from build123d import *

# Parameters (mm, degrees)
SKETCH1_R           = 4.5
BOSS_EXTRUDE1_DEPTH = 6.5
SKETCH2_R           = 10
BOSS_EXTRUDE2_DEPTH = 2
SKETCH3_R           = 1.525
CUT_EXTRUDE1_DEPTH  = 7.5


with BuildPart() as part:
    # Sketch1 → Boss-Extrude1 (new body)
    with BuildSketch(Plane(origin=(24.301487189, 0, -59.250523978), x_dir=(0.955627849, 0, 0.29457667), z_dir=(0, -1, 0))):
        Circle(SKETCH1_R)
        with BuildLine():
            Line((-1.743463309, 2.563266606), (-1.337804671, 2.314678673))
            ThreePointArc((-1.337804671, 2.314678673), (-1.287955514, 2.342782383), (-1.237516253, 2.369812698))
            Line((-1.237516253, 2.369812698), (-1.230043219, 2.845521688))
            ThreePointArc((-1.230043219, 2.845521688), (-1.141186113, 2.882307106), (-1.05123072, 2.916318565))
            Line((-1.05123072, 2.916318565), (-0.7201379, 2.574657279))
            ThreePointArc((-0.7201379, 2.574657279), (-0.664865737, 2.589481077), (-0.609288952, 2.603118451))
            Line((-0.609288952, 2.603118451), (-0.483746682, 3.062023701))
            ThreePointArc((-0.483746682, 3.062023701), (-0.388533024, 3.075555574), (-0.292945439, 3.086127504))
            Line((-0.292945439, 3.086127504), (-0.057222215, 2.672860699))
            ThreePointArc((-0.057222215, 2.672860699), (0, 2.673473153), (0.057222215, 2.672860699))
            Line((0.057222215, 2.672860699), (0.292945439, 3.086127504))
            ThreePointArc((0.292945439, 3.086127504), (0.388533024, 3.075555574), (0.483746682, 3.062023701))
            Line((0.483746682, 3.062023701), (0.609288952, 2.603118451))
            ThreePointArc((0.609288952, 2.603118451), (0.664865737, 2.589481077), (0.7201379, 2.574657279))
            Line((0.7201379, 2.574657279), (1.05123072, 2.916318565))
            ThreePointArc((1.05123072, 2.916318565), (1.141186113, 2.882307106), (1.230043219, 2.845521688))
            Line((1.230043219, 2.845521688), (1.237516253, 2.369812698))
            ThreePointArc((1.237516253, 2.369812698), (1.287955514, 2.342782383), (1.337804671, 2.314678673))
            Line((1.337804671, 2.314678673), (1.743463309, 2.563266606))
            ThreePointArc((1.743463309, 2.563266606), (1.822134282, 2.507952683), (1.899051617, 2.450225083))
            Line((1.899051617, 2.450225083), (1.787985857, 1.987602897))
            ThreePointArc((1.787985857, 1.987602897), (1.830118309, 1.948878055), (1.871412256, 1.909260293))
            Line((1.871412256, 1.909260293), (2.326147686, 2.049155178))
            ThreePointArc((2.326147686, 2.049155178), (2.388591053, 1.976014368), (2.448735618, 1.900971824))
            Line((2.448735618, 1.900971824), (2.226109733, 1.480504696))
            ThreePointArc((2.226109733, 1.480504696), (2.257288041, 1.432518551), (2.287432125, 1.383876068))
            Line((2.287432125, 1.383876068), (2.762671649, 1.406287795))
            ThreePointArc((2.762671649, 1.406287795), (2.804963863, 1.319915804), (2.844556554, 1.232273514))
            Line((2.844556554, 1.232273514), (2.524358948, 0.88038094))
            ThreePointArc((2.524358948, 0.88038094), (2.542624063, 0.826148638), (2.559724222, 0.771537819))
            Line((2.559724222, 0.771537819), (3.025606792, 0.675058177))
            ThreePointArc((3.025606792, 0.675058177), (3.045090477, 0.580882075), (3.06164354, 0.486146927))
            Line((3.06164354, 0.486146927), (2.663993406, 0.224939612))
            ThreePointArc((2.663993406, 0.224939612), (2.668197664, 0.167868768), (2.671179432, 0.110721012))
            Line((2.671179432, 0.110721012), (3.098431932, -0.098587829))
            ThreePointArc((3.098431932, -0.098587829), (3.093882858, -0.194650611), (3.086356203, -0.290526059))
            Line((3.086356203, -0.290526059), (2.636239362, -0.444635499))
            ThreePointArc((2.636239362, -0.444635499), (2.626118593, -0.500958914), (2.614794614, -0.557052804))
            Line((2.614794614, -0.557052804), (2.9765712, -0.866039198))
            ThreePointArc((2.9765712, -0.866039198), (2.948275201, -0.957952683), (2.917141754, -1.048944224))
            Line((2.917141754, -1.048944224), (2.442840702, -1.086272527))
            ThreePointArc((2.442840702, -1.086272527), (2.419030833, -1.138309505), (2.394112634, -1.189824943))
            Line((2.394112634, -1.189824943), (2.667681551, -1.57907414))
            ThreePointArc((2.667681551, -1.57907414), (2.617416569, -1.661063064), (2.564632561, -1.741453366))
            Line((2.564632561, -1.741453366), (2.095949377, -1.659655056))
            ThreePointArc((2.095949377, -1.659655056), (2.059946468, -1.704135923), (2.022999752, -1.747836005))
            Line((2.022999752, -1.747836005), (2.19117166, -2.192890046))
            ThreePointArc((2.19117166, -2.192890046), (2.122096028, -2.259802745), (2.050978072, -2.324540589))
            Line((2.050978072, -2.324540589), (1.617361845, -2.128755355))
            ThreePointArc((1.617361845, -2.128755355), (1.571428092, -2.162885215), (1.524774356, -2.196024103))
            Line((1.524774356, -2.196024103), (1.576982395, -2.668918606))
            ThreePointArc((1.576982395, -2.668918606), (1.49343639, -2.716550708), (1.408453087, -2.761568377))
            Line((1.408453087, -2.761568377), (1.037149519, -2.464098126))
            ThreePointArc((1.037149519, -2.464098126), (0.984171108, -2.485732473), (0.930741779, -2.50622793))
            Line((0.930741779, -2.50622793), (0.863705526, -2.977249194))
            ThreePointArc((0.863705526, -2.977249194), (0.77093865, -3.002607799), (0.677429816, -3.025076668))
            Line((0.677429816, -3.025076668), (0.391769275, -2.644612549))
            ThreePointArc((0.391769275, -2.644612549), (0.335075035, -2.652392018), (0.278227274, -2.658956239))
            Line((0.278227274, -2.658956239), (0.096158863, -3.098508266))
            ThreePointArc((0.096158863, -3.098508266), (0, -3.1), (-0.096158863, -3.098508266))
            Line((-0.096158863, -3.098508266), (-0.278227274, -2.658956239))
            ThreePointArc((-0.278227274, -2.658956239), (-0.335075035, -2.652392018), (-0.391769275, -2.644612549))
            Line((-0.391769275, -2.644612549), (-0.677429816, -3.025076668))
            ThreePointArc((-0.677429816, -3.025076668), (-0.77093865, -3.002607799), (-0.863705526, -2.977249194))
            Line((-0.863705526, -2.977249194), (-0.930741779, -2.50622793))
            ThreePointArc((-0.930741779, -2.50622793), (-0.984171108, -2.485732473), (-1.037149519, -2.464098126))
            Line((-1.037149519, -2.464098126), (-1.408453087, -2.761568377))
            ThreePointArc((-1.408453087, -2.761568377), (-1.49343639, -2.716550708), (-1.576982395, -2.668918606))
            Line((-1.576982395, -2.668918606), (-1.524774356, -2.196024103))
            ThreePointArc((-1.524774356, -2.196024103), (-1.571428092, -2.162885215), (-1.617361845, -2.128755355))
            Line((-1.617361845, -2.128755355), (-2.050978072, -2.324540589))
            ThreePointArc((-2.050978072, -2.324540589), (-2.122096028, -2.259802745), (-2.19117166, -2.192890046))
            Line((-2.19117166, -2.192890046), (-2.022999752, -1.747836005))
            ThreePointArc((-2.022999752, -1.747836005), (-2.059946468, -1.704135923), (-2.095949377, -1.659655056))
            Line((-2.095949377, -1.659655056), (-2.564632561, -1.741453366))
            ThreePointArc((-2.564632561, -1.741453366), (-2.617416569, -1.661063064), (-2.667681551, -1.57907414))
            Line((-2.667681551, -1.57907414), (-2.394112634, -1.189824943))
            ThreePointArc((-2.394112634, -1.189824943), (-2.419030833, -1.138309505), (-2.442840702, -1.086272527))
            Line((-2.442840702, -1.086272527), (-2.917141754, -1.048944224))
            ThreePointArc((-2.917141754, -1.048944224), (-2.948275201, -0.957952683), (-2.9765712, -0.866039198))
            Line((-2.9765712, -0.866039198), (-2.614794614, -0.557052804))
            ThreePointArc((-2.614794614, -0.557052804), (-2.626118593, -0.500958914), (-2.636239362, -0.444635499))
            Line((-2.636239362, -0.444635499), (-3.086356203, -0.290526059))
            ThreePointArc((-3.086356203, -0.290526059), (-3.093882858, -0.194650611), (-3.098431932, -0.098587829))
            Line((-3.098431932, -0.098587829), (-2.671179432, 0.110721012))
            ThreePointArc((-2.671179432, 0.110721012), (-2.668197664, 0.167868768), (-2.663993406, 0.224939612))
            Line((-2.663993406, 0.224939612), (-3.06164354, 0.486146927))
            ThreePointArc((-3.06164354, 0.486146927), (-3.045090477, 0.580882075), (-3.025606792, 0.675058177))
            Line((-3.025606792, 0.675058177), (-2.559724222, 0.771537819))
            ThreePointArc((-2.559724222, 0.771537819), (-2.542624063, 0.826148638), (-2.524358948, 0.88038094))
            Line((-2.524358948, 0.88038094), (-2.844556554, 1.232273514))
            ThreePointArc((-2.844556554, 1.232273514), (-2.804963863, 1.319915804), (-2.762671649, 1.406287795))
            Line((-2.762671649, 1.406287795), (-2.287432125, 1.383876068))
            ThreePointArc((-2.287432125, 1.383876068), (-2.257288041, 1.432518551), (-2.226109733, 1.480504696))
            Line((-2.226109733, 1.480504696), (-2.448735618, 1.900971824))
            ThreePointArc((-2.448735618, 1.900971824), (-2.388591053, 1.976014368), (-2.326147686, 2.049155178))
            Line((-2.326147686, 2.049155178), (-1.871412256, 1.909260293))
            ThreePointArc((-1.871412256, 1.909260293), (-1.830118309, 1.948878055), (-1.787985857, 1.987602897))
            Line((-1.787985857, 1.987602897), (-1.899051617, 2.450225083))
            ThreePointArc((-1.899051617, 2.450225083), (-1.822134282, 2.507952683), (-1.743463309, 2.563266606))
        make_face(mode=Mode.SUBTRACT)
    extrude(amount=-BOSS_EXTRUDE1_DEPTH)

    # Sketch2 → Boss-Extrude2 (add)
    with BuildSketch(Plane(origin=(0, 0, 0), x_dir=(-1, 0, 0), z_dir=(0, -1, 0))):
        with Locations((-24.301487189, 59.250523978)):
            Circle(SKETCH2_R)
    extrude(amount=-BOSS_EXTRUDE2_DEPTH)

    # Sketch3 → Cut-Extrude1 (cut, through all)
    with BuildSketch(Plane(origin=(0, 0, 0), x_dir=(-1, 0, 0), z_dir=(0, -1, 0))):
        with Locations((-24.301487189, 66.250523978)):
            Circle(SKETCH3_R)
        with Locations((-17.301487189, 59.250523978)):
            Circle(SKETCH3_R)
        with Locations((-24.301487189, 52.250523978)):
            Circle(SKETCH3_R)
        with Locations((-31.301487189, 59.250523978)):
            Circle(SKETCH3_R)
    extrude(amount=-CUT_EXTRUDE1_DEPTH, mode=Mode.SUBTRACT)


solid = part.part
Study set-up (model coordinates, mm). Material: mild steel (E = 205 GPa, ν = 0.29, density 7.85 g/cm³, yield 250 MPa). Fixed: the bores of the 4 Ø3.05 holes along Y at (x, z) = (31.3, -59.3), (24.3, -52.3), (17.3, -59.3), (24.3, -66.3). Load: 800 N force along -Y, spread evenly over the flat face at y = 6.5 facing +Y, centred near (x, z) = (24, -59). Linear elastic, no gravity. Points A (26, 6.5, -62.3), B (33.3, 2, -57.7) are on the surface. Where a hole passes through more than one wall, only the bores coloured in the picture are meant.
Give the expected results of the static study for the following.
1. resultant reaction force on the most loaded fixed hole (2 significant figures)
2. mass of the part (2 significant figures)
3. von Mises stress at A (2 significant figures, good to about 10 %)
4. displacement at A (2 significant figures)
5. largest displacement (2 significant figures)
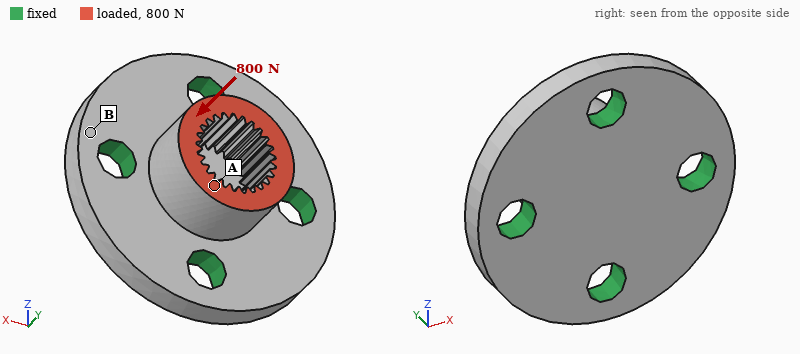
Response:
210 N
5.8 g
22 MPa
1.3 µm
1.3 µm
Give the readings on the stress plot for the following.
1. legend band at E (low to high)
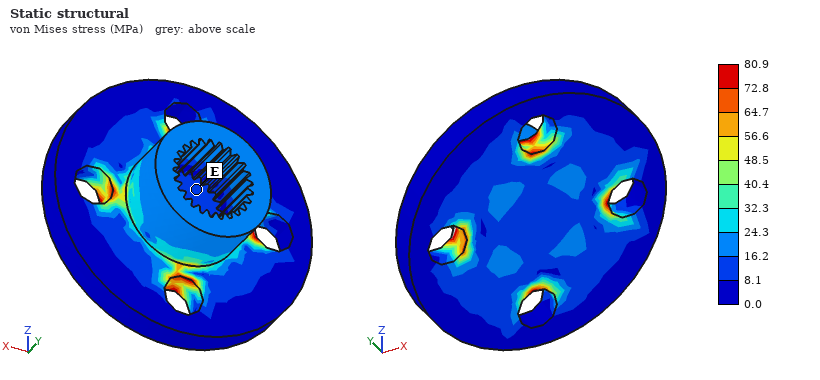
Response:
8.1 to 16.2 MPa
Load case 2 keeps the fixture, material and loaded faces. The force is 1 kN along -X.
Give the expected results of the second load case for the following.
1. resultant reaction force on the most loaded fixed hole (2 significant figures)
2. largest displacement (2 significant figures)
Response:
560 N
8.1 µm
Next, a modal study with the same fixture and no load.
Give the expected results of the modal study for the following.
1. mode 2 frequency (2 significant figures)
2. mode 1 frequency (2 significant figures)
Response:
78 kHz
78 kHz
